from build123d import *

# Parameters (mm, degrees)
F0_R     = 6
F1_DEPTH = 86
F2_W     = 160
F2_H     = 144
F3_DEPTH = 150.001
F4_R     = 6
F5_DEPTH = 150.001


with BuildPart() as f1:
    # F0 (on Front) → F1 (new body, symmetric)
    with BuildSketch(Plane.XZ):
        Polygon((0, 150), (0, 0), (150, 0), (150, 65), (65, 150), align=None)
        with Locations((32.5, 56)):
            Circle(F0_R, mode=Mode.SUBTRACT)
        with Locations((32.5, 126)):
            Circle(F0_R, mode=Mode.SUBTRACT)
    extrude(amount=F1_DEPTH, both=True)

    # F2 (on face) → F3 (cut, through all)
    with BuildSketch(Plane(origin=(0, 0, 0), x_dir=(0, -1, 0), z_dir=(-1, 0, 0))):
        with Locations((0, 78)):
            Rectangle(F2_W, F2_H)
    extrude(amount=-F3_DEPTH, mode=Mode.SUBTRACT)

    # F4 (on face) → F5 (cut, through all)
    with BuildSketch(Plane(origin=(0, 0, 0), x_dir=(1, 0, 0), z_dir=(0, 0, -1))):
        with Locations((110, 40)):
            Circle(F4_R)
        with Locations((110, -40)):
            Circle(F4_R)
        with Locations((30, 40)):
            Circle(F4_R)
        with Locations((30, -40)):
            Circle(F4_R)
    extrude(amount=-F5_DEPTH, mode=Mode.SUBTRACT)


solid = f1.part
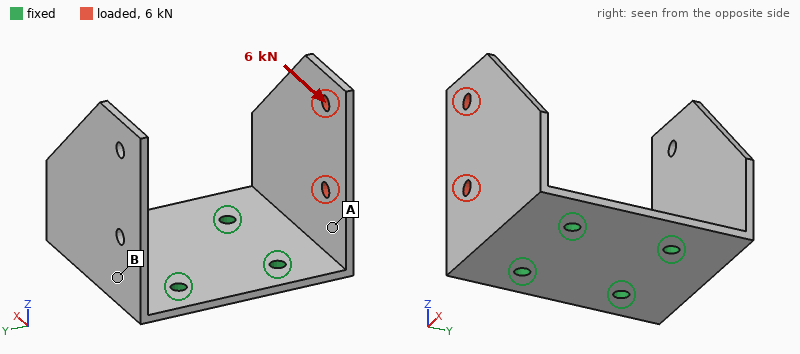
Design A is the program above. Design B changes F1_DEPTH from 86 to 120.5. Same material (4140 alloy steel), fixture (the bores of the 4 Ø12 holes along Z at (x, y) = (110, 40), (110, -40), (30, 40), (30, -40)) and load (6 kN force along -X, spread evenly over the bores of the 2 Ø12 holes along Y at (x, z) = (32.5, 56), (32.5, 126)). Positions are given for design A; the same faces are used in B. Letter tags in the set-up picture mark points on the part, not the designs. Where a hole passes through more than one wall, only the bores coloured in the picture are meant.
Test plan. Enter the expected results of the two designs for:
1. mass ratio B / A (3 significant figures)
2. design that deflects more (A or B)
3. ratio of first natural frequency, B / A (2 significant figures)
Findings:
4.53
A
0.46
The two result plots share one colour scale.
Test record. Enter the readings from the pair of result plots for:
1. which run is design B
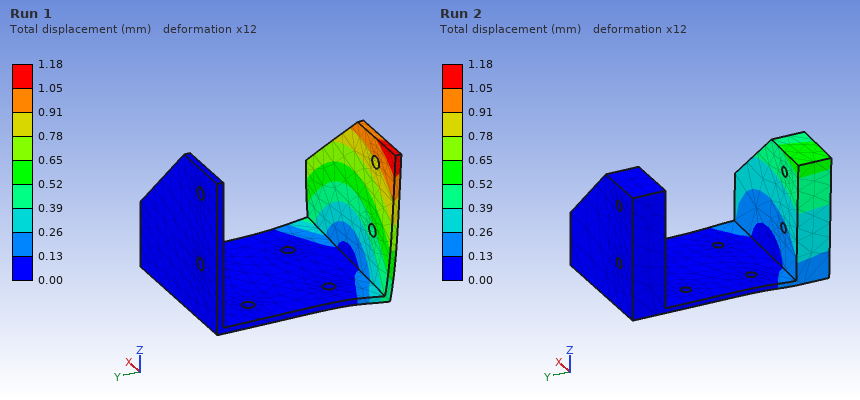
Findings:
Run 2
